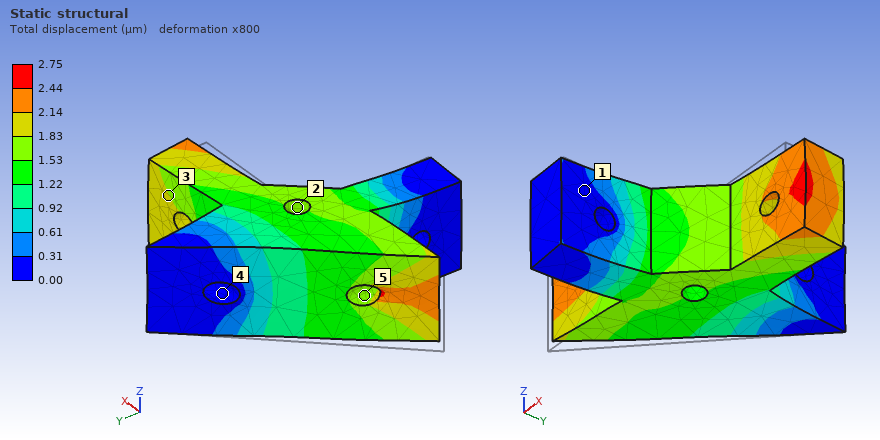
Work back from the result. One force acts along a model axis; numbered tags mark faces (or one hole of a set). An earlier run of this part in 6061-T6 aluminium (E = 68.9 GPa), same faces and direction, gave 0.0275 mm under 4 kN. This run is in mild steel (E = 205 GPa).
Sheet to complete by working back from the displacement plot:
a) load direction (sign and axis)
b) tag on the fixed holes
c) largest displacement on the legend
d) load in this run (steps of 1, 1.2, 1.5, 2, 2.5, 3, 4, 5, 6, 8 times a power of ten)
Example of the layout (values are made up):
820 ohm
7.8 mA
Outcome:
+X
4
2.75 µm
1.2 kN
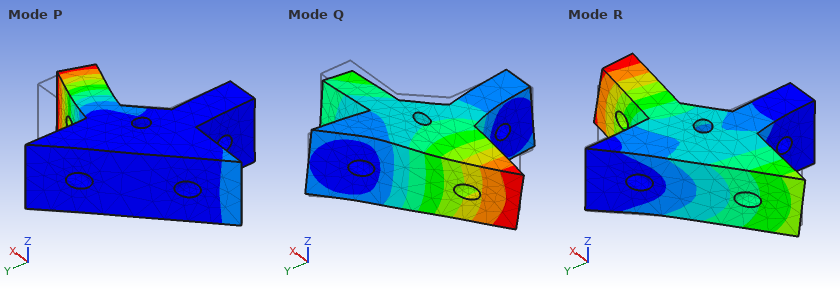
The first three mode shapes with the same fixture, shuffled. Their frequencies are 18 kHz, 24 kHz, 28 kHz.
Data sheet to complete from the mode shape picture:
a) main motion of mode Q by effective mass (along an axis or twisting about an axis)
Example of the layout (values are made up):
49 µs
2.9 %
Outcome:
along Z
